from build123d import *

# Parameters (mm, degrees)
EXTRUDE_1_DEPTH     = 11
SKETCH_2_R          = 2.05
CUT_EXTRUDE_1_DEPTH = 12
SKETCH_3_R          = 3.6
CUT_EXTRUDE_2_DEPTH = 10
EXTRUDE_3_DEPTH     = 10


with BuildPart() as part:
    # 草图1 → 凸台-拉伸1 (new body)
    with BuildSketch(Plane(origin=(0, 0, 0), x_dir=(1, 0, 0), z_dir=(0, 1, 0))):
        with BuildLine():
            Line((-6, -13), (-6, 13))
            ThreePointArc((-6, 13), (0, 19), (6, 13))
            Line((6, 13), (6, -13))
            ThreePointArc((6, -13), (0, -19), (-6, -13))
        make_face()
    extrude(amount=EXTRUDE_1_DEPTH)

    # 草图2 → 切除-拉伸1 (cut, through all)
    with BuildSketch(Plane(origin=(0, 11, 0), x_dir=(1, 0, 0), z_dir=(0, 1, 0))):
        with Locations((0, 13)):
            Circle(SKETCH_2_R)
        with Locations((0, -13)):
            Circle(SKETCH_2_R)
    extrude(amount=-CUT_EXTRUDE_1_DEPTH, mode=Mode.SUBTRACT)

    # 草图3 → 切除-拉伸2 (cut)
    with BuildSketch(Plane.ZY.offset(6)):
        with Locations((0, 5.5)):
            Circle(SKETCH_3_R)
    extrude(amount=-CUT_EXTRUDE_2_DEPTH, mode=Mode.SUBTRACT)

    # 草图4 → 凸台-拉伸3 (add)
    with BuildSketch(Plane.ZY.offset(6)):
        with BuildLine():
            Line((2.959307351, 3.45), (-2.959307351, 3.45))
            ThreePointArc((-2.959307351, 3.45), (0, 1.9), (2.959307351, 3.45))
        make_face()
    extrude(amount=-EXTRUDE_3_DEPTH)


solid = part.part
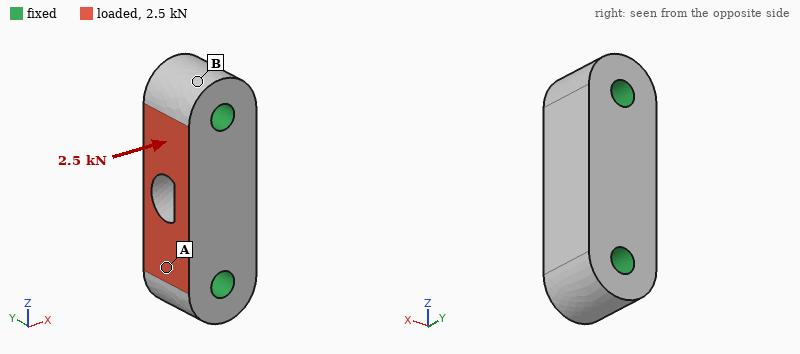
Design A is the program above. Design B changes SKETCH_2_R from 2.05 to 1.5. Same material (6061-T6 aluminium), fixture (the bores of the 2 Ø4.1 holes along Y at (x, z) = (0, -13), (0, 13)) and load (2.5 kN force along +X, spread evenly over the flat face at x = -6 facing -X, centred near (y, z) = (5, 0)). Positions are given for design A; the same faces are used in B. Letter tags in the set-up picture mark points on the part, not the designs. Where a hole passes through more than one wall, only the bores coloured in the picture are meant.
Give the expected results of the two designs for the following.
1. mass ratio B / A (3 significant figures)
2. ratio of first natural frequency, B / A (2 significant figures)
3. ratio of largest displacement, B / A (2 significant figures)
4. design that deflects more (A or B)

1.03
0.86
1.2
B
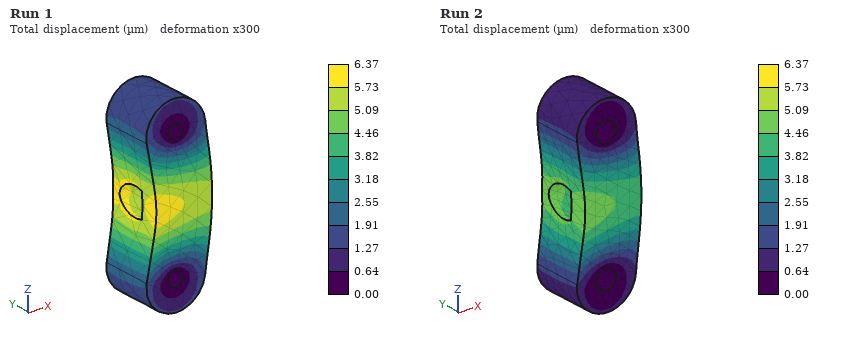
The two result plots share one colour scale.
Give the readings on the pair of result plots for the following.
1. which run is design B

Run 1
